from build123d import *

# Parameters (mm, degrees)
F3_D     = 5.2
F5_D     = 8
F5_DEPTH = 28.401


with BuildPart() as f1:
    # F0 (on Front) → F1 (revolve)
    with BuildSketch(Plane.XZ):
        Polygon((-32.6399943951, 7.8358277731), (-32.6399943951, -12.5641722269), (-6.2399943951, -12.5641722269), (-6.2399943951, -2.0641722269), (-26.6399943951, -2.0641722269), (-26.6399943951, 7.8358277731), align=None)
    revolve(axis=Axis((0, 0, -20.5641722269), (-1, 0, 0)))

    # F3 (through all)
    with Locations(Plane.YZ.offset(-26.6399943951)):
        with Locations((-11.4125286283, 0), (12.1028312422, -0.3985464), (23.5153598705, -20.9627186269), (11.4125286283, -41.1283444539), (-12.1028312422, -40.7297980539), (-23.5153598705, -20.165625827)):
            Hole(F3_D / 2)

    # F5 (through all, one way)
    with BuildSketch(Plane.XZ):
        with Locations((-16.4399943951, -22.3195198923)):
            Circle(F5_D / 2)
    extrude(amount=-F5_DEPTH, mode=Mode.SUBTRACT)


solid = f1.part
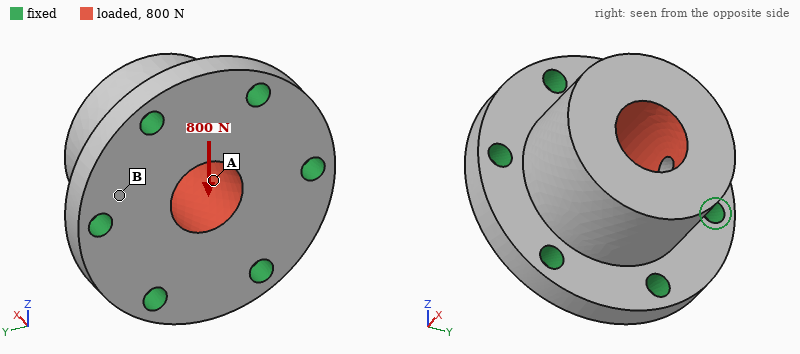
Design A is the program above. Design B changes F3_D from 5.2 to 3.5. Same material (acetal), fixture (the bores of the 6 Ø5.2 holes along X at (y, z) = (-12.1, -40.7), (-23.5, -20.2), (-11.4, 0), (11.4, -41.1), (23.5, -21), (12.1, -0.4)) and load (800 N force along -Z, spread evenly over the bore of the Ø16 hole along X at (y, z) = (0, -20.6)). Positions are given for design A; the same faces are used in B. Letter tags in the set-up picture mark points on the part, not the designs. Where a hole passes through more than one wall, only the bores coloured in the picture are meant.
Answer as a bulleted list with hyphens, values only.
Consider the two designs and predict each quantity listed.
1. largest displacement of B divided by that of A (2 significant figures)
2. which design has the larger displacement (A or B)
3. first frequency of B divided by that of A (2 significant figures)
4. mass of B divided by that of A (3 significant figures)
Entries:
- 1.1
- B
- 0.92
- 1.01
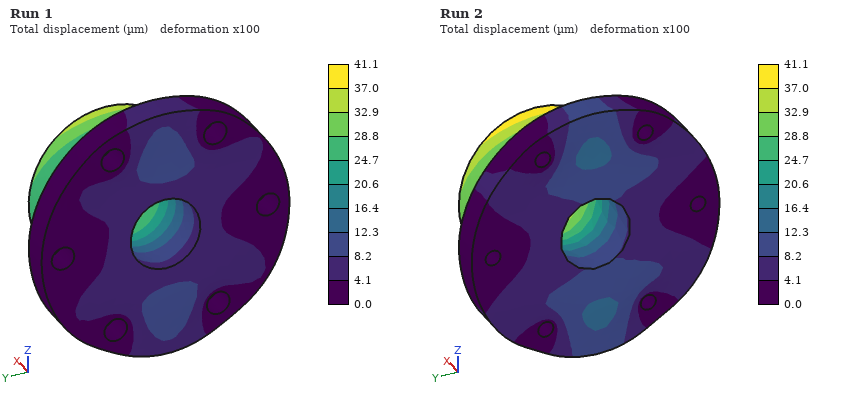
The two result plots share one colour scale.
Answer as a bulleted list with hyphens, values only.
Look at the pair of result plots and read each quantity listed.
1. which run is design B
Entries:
- Run 2
